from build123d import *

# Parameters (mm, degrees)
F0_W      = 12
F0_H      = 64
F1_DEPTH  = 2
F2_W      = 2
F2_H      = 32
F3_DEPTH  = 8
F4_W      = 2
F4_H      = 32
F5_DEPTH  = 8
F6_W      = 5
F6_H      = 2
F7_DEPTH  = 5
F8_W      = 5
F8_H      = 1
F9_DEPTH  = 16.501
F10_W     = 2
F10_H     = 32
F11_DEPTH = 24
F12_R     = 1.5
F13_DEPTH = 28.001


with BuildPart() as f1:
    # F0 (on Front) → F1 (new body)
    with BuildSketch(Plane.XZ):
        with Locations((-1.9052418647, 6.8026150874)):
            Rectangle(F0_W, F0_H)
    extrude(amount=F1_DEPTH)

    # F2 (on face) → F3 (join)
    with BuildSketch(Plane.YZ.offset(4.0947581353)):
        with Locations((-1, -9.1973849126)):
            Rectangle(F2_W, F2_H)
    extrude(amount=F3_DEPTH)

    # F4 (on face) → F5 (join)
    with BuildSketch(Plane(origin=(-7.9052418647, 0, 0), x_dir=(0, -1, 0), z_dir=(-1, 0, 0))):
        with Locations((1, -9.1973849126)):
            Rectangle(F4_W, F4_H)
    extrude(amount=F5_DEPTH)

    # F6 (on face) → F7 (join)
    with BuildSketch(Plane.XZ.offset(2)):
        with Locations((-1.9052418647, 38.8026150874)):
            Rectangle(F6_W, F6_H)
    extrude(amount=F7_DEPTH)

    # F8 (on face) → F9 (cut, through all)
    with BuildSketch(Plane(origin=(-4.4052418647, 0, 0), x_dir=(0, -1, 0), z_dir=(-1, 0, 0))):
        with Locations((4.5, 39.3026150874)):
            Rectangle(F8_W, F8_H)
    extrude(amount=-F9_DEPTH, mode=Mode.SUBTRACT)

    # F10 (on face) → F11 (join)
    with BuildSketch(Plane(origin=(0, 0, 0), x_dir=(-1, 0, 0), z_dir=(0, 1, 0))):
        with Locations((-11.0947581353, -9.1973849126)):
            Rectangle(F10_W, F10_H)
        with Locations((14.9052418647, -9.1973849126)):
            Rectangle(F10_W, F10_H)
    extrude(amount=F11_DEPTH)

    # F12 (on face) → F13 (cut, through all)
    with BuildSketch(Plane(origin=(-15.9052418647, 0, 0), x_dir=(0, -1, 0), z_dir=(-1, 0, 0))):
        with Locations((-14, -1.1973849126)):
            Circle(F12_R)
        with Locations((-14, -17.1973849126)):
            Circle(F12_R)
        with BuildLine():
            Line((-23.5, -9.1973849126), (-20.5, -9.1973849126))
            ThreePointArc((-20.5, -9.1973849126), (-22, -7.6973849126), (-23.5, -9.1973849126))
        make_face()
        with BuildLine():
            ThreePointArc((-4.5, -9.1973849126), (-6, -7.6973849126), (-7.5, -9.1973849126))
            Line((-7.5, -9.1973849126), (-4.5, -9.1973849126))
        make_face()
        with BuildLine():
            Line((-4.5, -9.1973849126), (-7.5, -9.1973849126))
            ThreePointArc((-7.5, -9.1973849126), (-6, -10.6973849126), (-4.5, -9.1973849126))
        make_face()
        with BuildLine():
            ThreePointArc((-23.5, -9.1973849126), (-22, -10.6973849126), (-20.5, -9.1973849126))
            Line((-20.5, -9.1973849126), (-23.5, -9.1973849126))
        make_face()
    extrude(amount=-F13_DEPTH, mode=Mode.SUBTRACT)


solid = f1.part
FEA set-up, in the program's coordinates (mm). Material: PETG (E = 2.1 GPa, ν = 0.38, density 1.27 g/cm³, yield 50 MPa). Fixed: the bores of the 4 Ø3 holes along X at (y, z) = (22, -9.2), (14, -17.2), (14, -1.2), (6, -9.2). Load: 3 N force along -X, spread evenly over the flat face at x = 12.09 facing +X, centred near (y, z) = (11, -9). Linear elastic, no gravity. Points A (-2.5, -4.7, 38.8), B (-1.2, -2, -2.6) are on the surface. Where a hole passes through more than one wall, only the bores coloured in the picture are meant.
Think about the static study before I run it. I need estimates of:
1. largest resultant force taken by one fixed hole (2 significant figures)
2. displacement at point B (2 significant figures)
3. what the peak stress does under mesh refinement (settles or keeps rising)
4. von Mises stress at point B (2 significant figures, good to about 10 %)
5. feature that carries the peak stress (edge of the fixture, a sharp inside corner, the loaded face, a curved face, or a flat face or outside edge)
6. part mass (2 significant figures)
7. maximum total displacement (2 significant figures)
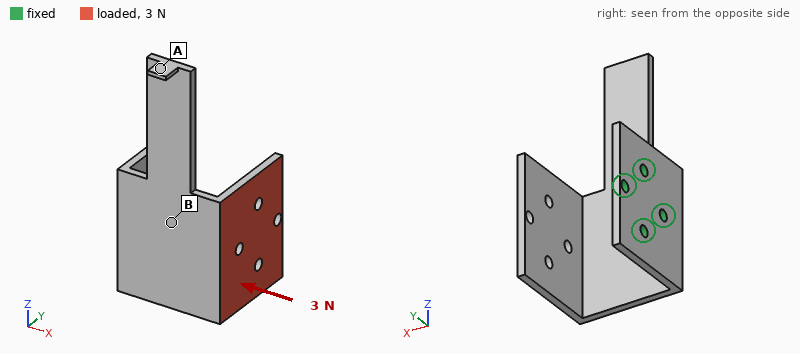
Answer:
1.1 N
0.11 mm
keeps rising
1.3 MPa
a sharp inside corner
7.0 g
0.70 mm
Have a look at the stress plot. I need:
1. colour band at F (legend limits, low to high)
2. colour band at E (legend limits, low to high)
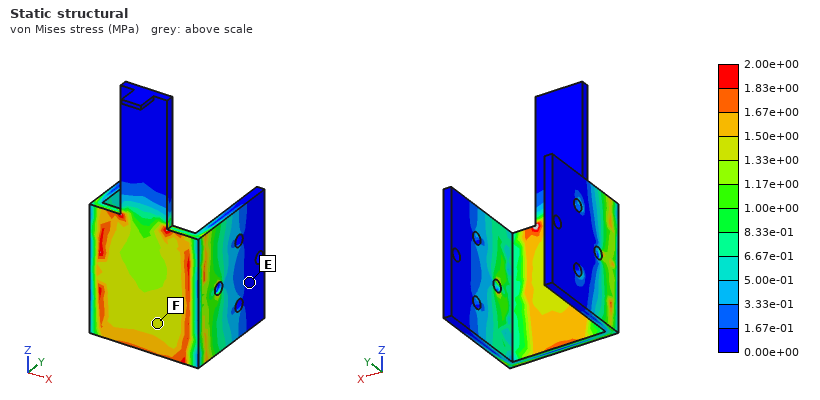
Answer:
1.33e+00 to 1.50e+00 MPa
0.00e+00 to 1.67e-01 MPa
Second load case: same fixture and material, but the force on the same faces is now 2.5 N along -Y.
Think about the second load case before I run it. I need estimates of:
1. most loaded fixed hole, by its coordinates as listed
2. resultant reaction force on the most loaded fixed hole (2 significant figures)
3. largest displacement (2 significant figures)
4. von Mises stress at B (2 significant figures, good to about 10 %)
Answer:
(6, -9.2)
5.0 N
0.86 mm
1.2 MPa
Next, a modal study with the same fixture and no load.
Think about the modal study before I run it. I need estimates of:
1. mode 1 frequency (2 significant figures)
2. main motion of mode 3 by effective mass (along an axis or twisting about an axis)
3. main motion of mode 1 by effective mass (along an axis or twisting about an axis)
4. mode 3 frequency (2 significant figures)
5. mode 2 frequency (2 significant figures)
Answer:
180 Hz
along Z
along Y
310 Hz
220 Hz
